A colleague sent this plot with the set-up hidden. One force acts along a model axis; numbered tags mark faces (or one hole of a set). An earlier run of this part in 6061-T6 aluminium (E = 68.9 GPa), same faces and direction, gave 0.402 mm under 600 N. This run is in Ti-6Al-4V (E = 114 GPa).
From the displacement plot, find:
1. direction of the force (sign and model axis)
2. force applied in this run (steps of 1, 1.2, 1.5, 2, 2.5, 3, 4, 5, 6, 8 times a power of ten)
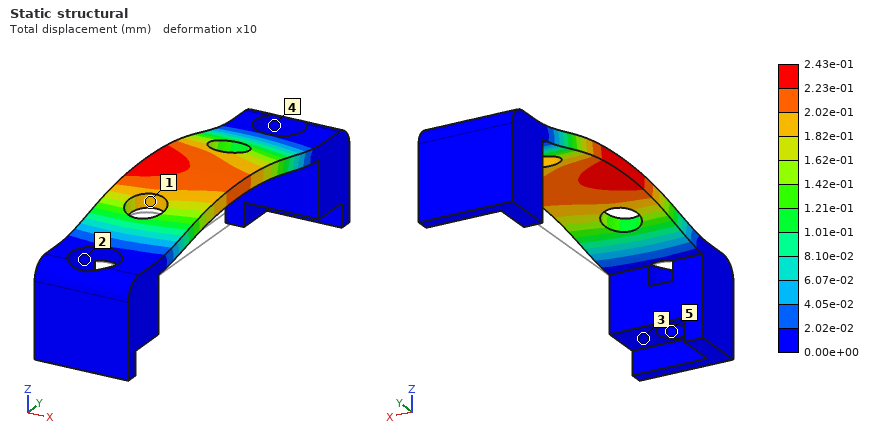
+Z
600 N
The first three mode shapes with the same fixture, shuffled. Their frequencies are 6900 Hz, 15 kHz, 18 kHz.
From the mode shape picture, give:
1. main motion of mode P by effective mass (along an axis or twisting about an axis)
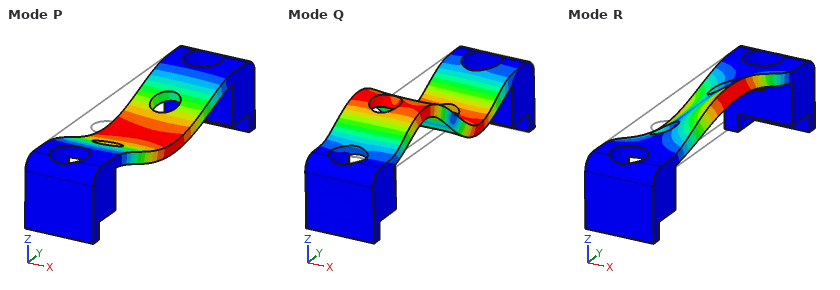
along Z
